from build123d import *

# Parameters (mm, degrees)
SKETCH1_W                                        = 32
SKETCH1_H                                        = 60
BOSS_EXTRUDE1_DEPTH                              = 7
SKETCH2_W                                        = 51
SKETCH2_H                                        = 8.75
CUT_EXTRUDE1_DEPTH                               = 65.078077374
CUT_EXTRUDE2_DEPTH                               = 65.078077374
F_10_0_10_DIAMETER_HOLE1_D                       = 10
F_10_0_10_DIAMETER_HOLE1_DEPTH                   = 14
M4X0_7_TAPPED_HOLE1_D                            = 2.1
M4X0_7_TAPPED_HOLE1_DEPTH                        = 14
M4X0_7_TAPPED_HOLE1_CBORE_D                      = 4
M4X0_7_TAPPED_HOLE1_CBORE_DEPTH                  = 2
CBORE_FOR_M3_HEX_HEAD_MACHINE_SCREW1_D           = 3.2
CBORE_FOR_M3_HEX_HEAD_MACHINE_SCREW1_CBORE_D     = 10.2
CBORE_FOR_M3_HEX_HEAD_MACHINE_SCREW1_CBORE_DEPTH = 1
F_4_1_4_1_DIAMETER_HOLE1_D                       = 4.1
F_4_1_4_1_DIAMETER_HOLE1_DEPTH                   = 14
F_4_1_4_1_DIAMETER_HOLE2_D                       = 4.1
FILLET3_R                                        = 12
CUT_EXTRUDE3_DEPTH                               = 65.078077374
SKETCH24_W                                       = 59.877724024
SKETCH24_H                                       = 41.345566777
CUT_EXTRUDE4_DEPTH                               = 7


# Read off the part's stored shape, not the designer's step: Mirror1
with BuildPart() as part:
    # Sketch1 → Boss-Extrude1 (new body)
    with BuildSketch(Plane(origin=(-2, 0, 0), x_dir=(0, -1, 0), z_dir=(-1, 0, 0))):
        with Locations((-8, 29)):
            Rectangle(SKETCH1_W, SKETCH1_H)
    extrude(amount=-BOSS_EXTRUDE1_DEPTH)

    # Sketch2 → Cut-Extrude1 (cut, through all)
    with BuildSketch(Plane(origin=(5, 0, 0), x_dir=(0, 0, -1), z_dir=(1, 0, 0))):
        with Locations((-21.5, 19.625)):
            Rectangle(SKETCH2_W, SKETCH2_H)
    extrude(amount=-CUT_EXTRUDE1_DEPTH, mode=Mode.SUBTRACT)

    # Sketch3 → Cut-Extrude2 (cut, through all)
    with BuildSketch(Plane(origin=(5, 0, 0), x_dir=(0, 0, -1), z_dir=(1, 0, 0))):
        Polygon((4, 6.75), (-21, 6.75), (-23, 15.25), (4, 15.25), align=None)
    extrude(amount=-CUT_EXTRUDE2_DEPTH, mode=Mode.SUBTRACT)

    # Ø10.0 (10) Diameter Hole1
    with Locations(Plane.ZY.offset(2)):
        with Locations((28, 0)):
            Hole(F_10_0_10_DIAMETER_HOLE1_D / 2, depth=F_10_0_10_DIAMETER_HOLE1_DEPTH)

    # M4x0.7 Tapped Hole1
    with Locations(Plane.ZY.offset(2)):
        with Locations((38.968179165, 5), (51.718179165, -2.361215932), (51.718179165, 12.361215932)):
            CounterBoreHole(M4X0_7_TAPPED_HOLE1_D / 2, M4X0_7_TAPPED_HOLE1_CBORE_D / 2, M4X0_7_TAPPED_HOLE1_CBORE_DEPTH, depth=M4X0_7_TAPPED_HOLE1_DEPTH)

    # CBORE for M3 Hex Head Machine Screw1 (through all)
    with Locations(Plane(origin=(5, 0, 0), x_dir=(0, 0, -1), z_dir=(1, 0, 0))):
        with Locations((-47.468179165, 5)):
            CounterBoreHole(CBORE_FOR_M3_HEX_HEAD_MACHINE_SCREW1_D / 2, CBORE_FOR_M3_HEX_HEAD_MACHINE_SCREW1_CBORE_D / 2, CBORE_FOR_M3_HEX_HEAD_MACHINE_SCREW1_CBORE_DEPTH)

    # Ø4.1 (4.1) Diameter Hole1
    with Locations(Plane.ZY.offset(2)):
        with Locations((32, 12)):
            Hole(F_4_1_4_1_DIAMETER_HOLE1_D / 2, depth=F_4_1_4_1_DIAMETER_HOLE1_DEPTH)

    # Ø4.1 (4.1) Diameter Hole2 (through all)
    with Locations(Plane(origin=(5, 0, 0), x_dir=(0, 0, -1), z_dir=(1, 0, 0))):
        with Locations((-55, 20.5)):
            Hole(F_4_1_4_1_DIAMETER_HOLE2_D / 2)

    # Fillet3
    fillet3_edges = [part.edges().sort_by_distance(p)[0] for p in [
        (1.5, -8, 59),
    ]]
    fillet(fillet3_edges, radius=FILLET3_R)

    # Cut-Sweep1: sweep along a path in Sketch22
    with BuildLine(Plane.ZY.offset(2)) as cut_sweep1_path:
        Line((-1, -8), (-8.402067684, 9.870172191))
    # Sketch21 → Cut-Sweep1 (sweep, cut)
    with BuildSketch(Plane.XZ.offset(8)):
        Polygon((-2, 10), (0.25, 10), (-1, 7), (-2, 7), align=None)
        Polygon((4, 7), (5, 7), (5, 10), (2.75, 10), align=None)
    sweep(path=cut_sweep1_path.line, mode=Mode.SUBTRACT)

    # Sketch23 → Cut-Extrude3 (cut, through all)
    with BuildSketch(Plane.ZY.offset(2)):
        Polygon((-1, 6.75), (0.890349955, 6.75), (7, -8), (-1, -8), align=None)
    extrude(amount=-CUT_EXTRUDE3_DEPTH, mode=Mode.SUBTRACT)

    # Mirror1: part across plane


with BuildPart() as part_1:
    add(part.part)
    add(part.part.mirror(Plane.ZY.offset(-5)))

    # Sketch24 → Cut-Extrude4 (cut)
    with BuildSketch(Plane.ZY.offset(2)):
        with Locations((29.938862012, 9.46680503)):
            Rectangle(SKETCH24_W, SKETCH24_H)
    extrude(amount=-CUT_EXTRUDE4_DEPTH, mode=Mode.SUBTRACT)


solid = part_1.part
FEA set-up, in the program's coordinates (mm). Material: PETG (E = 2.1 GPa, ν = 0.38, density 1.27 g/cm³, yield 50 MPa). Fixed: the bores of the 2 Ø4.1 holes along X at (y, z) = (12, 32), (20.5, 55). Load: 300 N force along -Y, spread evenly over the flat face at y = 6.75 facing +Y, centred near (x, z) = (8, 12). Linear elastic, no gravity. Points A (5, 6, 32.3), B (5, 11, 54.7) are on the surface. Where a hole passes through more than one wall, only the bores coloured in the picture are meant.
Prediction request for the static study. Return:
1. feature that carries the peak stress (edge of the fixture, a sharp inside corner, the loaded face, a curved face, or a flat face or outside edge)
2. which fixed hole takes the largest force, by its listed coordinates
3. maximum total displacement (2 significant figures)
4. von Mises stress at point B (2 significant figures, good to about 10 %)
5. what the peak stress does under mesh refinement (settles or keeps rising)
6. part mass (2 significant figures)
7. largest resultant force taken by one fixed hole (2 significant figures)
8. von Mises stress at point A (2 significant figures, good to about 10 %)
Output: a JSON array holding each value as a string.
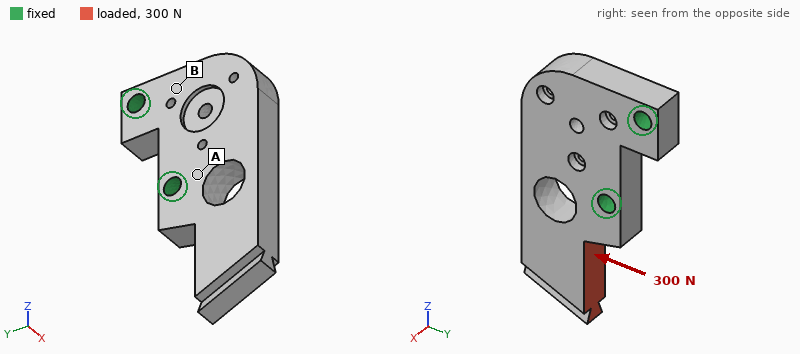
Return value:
["edge of the fixture", "(12, 32)", "0.54 mm", "2.9 MPa", "keeps rising", "9.2 g", "530 N", "7.0 MPa"]
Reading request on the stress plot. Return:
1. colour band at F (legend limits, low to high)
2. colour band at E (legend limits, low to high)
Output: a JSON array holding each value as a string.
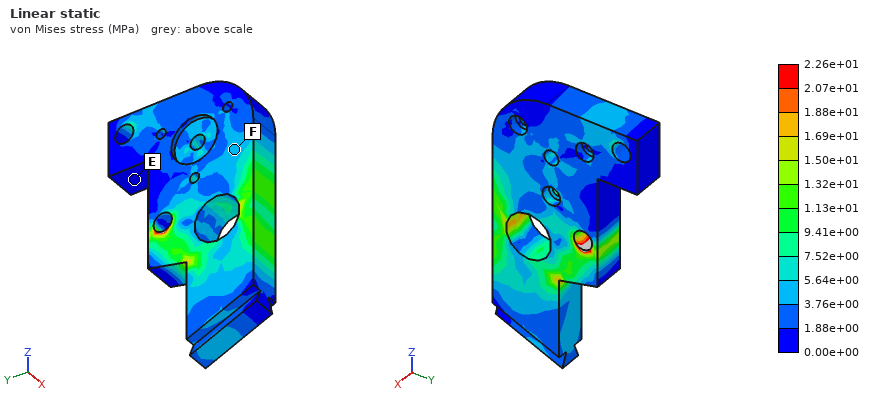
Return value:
["3.76e+00 to 5.64e+00 MPa", "0.00e+00 to 1.88e+00 MPa"]
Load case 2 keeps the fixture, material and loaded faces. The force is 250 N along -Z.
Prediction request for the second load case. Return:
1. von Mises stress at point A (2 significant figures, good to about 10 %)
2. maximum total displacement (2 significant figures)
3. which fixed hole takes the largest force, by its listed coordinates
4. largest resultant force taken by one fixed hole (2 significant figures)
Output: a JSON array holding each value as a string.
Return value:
["4.6 MPa", "0.17 mm", "(12, 32)", "230 N"]
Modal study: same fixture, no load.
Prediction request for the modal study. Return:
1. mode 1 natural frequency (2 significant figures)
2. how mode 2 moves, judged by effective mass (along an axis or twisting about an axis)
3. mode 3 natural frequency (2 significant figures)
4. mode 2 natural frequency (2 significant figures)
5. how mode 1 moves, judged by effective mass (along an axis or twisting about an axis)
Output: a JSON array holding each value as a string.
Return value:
["1400 Hz", "along X", "3000 Hz", "2300 Hz", "along X"]
